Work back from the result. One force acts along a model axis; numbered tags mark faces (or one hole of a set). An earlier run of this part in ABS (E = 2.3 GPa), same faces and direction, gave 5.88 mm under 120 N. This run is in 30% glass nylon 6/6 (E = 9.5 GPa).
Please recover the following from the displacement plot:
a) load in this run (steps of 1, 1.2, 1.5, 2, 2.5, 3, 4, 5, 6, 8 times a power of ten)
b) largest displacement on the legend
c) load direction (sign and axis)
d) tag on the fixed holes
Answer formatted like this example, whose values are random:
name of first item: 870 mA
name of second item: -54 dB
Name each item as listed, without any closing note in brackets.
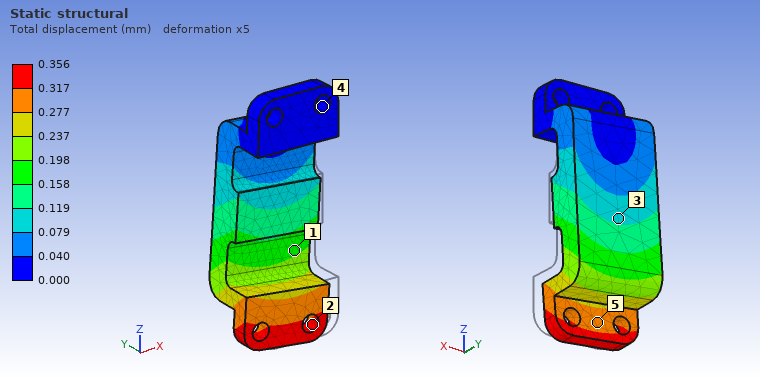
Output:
load in this run: 30 N
largest displacement on the legend: 0.356 mm
load direction: -X
tag on the fixed holes: 4
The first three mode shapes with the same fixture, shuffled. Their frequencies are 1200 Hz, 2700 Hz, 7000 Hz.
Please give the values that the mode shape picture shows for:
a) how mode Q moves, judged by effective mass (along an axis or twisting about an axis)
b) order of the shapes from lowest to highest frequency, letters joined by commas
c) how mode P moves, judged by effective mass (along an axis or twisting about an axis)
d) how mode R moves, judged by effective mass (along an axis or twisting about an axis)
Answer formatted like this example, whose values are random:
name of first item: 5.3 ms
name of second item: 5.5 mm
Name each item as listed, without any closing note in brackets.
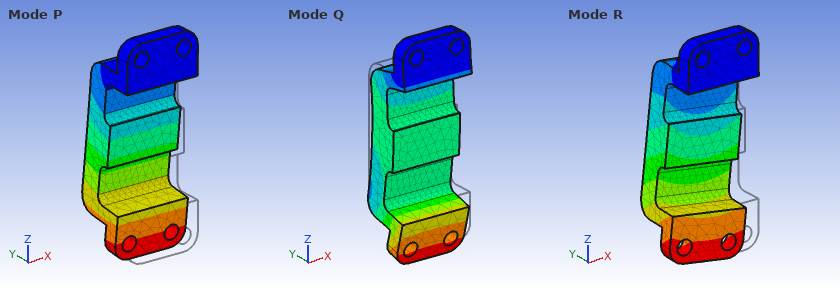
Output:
how mode Q moves, judged by effective mass: along Z
order of the shapes from lowest to highest frequency, letters joined by commas: P, R, Q
how mode P moves, judged by effective mass: along Y
how mode R moves, judged by effective mass: along X
